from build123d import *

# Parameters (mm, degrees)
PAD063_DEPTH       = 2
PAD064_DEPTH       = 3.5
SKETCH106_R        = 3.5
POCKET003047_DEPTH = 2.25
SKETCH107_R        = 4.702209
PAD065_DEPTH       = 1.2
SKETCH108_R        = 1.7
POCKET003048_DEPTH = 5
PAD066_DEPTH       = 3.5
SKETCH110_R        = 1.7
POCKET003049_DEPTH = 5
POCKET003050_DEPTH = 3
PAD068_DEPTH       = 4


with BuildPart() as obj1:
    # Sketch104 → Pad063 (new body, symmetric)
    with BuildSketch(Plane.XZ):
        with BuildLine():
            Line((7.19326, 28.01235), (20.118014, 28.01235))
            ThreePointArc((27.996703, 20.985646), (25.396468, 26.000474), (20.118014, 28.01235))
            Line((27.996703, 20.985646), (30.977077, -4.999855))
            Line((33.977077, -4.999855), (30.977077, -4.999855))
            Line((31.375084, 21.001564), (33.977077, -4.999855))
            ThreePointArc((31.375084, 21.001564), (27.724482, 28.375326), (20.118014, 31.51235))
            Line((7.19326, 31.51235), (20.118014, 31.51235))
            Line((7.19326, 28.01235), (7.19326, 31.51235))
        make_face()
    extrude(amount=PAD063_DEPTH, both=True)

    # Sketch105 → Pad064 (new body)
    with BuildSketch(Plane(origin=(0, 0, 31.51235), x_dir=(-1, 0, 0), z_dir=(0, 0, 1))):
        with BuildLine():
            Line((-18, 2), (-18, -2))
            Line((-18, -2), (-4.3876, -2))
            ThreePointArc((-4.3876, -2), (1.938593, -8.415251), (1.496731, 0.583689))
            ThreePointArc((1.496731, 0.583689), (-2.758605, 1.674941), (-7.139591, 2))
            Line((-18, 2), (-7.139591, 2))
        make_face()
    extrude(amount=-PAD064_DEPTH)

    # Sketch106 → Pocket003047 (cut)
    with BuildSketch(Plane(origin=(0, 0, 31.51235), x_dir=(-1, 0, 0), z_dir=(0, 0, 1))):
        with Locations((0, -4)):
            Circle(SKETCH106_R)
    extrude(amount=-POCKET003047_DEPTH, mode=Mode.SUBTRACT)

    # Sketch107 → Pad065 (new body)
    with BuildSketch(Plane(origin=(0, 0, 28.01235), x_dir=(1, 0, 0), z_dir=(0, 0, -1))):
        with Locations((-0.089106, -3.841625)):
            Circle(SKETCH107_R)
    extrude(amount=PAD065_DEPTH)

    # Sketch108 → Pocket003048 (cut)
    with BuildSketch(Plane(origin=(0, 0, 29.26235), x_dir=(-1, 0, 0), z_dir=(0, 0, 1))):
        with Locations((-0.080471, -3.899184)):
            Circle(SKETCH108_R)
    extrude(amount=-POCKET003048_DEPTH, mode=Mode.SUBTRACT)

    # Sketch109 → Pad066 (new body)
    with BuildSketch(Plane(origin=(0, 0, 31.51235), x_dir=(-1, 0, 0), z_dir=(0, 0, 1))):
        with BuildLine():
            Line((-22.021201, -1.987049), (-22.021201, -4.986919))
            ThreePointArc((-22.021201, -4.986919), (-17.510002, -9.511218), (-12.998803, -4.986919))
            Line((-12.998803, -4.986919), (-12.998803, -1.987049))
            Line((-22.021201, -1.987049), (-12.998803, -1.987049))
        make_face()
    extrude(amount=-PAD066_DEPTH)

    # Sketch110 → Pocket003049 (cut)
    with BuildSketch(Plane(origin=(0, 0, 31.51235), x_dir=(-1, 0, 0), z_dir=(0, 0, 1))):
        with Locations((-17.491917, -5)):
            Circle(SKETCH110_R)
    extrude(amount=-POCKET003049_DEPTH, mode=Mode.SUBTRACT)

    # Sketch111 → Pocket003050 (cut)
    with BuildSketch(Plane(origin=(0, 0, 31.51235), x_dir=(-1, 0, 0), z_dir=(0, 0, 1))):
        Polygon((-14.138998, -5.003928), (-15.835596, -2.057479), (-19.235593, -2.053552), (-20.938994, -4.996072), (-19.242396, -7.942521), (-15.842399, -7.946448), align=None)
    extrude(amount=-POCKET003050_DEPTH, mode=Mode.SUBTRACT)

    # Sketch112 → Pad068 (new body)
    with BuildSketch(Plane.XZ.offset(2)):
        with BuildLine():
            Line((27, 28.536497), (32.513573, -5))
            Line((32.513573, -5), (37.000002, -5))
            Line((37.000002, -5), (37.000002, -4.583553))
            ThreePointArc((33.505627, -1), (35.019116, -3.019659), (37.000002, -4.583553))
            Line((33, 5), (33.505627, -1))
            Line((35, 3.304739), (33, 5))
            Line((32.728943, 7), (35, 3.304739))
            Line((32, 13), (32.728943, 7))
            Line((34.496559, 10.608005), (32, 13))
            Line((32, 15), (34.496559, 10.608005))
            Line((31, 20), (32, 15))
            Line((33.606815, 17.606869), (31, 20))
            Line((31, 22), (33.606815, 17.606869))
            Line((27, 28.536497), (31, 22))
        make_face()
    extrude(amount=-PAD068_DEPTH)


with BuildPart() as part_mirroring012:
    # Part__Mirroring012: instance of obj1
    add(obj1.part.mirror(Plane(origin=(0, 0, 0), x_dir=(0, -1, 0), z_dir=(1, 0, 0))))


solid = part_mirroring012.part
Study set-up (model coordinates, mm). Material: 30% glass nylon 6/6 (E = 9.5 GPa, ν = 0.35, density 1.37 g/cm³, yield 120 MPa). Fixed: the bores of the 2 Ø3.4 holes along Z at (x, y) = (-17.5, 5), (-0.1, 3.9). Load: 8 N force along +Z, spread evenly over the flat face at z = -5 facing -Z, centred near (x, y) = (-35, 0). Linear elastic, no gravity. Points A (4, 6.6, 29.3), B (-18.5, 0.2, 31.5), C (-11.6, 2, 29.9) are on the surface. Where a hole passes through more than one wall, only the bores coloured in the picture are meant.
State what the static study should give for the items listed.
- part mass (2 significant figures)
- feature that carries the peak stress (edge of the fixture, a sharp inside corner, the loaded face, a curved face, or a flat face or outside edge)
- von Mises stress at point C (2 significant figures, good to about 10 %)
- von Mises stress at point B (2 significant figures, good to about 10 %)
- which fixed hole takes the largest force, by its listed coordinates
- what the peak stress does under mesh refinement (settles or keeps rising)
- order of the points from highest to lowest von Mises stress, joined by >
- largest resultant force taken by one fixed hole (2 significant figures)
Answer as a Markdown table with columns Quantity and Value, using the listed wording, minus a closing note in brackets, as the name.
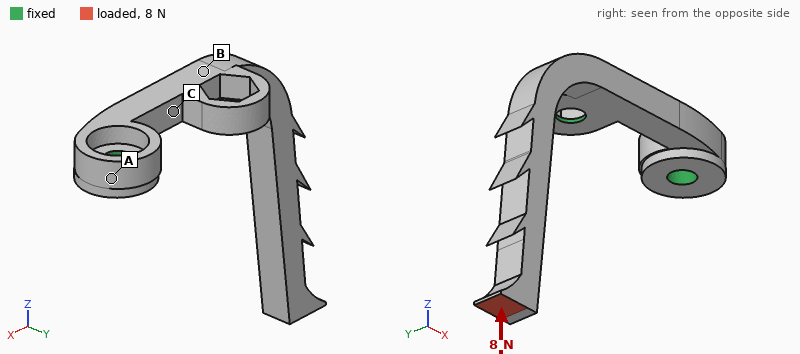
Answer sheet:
| Quantity | Value |
|---|---|
| part mass | 1.6 g |
| feature that carries the peak stress | edge of the fixture |
| von Mises stress at point C | 5.0 MPa |
| von Mises stress at point B | 13 MPa |
| which fixed hole takes the largest force, by its listed coordinates | (-17.5, 5) |
| what the peak stress does under mesh refinement | keeps rising |
| order of the points from highest to lowest von Mises stress, joined by > | B > C > A |
| largest resultant force taken by one fixed hole | 18 N |
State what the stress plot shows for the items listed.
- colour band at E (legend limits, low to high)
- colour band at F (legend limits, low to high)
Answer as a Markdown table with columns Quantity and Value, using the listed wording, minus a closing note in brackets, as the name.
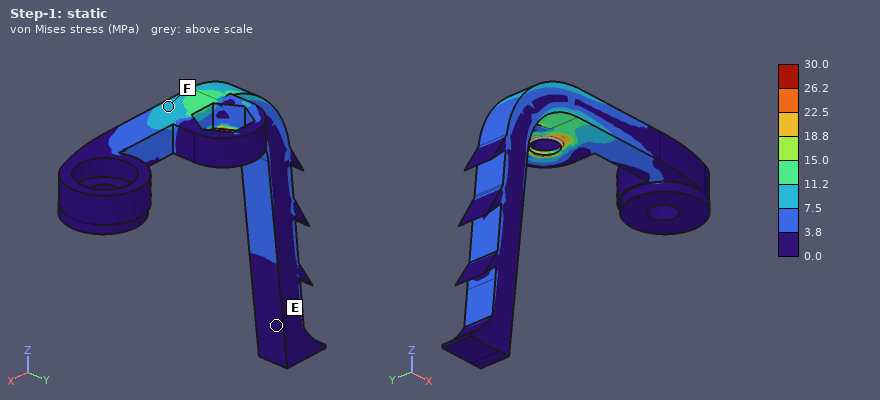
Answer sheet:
| Quantity | Value |
|---|---|
| colour band at E | 0.0 to 3.8 MPa |
| colour band at F | 7.5 to 11.2 MPa |
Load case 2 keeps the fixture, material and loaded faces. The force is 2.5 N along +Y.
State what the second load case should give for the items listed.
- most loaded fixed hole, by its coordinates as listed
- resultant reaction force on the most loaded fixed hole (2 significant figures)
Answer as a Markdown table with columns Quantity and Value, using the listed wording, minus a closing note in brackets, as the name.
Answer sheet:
| Quantity | Value |
|---|---|
| most loaded fixed hole, by its coordinates as listed | (-17.5, 5) |
| resultant reaction force on the most loaded fixed hole | 6.5 N |
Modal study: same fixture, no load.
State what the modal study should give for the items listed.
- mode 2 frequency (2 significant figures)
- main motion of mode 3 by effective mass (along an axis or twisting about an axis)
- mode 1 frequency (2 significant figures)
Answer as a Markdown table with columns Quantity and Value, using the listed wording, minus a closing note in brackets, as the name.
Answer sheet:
| Quantity | Value |
|---|---|
| mode 2 frequency | 760 Hz |
| main motion of mode 3 by effective mass | along Z |
| mode 1 frequency | 680 Hz |
